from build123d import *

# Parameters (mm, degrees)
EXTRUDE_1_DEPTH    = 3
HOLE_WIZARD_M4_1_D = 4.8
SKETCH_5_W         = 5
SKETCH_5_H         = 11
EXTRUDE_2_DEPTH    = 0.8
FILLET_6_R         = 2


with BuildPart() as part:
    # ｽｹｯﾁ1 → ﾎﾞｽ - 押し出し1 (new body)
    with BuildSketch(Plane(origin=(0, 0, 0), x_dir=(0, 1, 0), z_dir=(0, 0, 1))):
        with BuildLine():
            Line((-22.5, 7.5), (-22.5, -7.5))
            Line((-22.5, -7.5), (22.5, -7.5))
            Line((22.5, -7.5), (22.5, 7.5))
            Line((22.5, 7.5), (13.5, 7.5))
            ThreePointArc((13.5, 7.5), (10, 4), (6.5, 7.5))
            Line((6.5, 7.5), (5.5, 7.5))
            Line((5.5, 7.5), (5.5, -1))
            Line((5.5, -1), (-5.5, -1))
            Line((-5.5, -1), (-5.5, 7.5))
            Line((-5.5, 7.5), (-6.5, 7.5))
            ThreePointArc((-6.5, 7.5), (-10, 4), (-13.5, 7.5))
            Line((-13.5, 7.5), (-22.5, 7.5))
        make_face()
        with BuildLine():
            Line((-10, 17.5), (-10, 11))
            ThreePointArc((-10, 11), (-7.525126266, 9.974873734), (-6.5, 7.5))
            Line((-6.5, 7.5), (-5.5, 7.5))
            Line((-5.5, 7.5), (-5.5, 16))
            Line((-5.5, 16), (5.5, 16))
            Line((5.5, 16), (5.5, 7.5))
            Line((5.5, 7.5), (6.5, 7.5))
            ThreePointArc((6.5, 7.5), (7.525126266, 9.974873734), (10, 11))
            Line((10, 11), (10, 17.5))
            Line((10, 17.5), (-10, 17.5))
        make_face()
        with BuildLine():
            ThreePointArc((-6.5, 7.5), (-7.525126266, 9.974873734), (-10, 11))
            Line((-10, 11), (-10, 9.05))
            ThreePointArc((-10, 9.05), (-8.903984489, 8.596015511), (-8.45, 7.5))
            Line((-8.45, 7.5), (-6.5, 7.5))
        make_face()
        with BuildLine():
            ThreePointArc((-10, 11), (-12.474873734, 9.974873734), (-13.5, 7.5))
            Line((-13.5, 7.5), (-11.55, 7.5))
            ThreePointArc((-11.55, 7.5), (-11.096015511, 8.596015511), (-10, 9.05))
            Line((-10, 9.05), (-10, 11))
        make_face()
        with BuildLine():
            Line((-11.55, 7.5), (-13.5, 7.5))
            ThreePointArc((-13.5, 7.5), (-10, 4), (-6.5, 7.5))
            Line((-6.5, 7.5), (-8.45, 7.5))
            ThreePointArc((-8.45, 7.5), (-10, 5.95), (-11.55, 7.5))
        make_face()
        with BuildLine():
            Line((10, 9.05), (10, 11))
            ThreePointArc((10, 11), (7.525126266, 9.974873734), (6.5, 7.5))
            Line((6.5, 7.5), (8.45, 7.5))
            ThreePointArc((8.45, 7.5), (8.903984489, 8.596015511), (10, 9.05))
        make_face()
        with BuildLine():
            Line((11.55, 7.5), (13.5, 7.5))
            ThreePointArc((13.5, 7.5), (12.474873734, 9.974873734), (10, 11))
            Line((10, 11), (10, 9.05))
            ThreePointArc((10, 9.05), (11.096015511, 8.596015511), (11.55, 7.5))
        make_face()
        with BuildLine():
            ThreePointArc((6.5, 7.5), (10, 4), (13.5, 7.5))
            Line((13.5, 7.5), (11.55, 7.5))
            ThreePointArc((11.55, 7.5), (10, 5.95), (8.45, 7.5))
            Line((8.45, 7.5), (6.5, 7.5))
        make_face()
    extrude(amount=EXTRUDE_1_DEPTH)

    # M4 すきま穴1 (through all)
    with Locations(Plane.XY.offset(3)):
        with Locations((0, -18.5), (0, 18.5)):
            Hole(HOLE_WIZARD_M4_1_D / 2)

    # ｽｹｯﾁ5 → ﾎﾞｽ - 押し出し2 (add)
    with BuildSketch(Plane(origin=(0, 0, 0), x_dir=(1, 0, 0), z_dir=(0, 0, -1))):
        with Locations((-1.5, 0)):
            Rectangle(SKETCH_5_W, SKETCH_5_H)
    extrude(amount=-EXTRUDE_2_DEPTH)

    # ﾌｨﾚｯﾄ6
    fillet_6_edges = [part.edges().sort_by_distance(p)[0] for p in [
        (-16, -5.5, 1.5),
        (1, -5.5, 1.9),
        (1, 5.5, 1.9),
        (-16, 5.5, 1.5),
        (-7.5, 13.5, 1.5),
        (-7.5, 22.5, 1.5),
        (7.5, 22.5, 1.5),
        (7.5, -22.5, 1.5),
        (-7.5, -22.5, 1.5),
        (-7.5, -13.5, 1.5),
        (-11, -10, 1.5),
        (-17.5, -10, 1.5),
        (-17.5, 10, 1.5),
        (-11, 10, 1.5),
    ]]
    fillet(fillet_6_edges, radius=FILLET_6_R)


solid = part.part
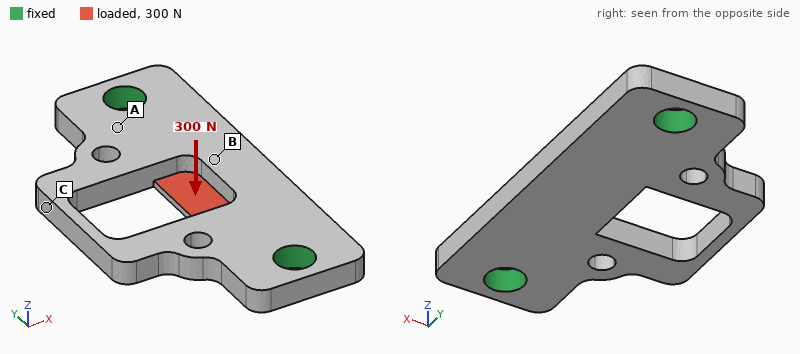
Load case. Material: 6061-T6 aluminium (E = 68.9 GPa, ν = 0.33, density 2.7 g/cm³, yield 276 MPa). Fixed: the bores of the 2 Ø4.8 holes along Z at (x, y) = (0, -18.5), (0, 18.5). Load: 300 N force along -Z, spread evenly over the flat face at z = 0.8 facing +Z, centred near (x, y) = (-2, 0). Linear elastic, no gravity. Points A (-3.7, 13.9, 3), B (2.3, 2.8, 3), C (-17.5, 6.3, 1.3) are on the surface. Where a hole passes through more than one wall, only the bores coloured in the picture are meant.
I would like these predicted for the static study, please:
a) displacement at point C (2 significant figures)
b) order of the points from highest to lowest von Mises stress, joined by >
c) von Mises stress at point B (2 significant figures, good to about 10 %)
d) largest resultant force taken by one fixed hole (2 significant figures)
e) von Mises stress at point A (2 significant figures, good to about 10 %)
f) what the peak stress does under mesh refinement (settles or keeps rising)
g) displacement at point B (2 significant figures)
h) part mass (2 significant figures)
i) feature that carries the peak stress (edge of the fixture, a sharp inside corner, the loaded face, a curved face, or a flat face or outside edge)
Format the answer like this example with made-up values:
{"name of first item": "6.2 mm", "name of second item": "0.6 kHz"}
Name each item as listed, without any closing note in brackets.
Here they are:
{"displacement at point C": "0.025 mm", "order of the points from highest to lowest von Mises stress, joined by >": "B > A > C", "von Mises stress at point B": "64 MPa", "largest resultant force taken by one fixed hole": "190 N", "von Mises stress at point A": "40 MPa", "what the peak stress does under mesh refinement": "keeps rising", "displacement at point B": "0.031 mm", "part mass": "5.4 g", "feature that carries the peak stress": "a sharp inside corner"}
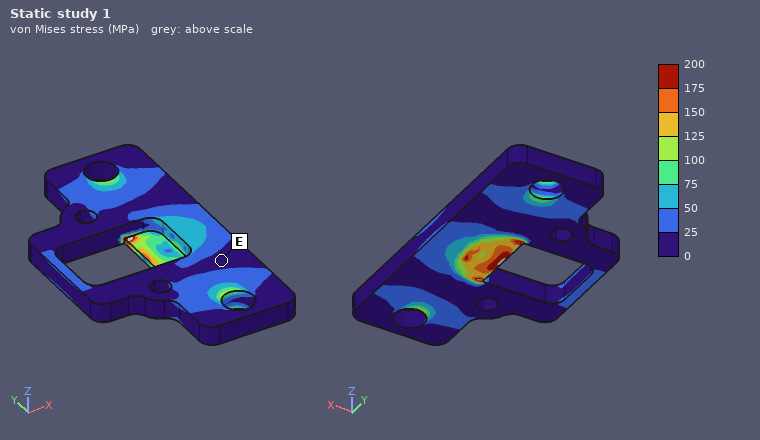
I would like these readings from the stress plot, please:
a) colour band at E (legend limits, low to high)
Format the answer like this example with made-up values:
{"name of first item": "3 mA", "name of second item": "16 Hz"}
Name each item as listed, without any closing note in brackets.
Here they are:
{"colour band at E": "0 to 25 MPa"}
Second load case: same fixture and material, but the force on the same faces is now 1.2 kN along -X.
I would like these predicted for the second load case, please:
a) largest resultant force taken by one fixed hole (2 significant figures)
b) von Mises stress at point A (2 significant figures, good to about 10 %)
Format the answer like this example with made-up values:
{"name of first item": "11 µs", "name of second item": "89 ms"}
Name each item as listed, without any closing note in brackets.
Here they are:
{"largest resultant force taken by one fixed hole": "650 N", "von Mises stress at point A": "32 MPa"}
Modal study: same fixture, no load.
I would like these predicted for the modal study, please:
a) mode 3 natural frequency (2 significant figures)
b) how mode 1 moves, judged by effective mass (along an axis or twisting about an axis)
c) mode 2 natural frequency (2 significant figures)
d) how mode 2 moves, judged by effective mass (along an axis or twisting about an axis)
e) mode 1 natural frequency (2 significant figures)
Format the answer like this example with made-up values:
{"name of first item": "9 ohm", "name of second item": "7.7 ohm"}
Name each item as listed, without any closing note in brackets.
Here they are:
{"mode 3 natural frequency": "15 kHz", "how mode 1 moves, judged by effective mass": "along Z", "mode 2 natural frequency": "13 kHz", "how mode 2 moves, judged by effective mass": "along Z", "mode 1 natural frequency": "7600 Hz"}
